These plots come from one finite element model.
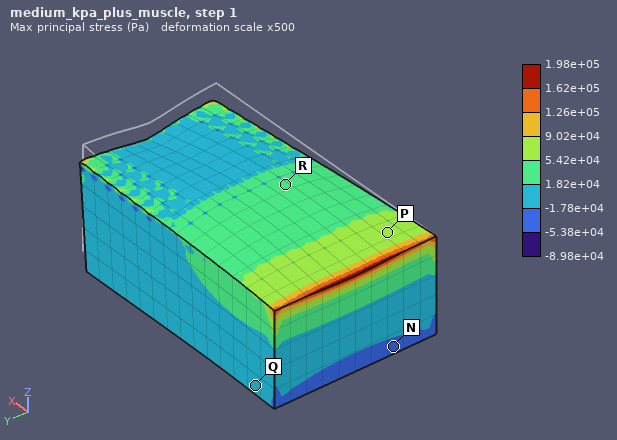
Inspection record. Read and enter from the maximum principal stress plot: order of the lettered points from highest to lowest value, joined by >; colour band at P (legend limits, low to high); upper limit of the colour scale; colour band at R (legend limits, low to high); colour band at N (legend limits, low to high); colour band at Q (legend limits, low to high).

P > R > Q > N
5.42e+04 to 9.02e+04 Pa
1.98e+05 Pa
1.82e+04 to 5.42e+04 Pa
-5.38e+04 to -1.78e+04 Pa
-1.78e+04 to 1.82e+04 Pa
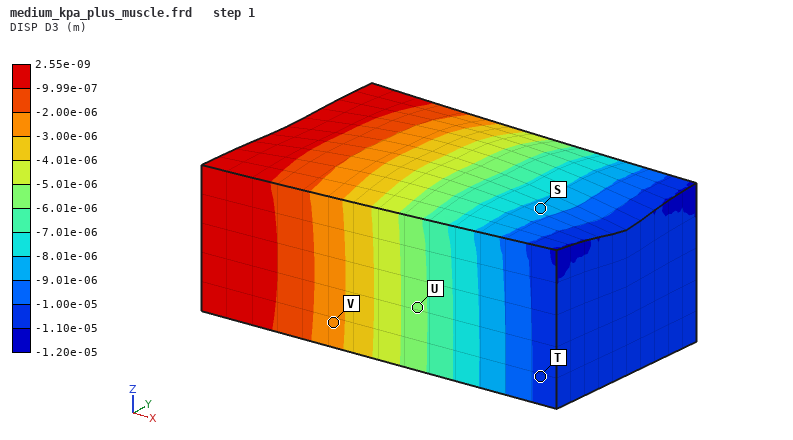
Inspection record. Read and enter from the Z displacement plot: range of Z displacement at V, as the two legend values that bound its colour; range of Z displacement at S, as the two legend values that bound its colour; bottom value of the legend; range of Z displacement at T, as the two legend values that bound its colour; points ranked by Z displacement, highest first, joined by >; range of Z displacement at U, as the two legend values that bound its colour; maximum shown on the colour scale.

-3.00e-06 to -2.00e-06 m
-9.01e-06 to -8.01e-06 m
-1.20e-05 m
-1.10e-05 to -1.00e-05 m
V > U > S > T
-6.01e-06 to -5.01e-06 m
2.55e-09 m
